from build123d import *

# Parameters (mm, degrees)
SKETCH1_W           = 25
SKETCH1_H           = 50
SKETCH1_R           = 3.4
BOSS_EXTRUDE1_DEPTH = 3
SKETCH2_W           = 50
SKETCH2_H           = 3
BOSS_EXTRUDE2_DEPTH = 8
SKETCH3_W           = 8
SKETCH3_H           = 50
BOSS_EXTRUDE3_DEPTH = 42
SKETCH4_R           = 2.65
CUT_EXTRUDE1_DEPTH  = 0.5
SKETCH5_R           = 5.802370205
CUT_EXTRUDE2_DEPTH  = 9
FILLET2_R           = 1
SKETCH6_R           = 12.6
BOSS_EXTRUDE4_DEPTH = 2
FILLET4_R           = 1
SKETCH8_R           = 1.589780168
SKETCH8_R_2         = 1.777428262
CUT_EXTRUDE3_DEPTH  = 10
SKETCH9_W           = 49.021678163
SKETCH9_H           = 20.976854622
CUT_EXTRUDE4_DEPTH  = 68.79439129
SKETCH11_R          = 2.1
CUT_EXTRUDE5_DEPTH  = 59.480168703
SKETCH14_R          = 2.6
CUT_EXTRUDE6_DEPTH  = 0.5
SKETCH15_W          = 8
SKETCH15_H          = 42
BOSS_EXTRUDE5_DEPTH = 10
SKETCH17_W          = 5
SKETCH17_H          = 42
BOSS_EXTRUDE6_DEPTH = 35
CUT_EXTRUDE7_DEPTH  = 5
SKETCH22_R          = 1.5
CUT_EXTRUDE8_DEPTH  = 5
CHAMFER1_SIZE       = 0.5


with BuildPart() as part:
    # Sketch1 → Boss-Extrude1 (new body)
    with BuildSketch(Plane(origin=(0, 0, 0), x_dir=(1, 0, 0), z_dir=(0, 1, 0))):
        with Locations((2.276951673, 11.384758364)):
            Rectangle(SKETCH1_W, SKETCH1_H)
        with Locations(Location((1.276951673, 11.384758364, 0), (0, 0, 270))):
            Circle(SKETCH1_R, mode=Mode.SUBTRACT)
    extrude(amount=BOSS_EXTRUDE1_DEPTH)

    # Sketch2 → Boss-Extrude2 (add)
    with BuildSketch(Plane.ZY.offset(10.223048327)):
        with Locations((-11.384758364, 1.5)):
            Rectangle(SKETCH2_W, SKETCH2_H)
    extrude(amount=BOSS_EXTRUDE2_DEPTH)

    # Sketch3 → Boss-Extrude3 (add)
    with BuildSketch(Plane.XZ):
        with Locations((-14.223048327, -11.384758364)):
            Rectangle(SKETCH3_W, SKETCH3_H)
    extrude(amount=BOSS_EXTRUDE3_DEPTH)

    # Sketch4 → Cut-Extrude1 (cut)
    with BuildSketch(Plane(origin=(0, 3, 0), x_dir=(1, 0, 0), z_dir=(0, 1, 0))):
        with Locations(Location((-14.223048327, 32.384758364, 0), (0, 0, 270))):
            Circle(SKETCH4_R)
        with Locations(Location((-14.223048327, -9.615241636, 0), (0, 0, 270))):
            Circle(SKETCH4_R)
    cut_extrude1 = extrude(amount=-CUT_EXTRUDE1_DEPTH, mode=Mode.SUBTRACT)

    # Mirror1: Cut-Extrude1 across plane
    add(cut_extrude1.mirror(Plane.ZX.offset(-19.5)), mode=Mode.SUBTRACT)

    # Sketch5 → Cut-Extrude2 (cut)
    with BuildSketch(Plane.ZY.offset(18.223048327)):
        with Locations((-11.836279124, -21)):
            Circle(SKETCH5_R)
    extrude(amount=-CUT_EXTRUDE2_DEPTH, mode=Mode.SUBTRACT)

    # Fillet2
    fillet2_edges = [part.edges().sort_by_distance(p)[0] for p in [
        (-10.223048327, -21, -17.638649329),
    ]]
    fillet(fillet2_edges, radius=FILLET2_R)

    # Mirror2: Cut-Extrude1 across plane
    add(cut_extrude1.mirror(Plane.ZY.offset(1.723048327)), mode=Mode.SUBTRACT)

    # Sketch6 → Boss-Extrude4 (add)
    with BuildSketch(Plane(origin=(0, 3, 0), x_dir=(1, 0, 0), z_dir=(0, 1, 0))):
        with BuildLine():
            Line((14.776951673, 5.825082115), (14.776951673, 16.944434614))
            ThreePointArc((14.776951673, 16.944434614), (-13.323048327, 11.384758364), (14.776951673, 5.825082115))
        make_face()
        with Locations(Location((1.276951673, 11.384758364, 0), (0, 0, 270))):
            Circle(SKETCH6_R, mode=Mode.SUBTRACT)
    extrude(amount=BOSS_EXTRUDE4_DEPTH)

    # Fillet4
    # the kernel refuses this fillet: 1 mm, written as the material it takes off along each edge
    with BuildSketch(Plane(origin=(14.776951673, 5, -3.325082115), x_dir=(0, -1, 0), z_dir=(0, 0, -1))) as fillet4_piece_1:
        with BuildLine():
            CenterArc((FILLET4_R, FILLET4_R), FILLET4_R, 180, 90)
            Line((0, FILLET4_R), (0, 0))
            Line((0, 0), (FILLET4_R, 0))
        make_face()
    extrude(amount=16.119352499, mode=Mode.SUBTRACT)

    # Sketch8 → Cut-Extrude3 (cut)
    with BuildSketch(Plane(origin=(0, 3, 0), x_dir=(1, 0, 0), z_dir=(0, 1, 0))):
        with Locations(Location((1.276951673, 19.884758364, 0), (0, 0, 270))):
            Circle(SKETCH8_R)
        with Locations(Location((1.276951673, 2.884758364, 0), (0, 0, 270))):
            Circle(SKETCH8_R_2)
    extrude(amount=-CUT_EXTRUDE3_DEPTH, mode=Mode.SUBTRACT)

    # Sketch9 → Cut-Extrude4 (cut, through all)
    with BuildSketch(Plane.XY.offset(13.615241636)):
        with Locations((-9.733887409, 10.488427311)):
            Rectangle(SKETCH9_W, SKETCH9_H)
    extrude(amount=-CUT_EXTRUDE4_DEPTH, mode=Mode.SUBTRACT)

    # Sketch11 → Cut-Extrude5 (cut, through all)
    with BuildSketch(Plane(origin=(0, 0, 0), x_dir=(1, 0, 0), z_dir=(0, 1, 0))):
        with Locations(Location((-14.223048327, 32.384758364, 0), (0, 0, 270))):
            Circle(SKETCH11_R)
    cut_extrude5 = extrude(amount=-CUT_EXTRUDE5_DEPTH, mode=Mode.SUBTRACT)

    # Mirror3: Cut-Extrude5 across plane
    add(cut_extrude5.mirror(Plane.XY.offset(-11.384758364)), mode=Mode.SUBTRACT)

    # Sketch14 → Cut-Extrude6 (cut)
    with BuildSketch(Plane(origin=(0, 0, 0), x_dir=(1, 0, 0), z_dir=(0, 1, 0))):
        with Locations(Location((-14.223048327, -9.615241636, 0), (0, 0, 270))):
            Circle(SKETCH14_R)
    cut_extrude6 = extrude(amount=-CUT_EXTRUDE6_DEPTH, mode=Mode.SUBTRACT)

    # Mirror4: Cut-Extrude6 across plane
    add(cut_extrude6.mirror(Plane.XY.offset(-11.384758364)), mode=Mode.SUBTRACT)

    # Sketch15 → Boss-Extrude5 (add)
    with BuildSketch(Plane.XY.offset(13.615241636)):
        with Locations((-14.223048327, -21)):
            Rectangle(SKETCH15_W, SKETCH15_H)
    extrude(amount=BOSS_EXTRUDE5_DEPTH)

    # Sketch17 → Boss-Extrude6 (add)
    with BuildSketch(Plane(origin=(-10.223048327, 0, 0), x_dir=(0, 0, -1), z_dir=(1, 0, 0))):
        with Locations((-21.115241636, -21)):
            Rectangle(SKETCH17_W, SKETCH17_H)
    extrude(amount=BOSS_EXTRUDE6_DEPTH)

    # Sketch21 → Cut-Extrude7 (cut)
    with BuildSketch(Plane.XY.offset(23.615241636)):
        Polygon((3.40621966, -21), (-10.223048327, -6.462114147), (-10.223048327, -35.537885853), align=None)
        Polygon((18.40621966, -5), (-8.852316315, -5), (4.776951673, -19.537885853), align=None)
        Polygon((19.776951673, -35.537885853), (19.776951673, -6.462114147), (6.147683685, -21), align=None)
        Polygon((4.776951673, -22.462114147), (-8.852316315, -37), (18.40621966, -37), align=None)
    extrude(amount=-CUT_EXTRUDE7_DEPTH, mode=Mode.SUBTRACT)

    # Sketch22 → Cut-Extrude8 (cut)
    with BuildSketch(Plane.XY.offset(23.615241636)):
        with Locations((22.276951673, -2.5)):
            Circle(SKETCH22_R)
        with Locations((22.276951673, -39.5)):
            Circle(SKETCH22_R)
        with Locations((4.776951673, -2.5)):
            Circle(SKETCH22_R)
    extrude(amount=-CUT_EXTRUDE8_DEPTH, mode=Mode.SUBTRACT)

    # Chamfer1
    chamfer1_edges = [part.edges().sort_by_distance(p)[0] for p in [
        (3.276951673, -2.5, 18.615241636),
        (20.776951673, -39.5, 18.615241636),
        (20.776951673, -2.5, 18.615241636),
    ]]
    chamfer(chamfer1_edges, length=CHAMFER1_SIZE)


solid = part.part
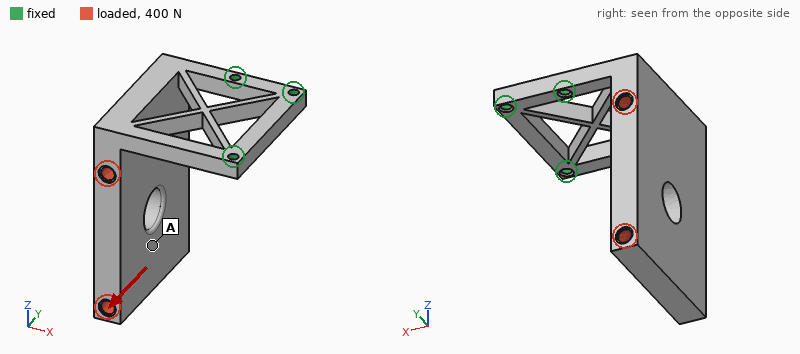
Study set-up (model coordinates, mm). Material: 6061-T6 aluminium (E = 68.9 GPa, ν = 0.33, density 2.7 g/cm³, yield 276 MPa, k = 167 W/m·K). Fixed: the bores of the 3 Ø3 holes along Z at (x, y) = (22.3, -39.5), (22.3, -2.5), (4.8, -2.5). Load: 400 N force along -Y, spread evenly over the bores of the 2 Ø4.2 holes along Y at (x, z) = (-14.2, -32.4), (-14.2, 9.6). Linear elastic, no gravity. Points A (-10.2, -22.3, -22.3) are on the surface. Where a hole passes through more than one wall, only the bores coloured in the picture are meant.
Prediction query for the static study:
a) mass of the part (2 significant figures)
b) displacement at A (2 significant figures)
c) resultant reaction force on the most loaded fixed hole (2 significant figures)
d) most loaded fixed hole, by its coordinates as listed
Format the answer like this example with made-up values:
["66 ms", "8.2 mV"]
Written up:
["58 g", "0.55 mm", "450 N", "(22.3, -39.5)"]
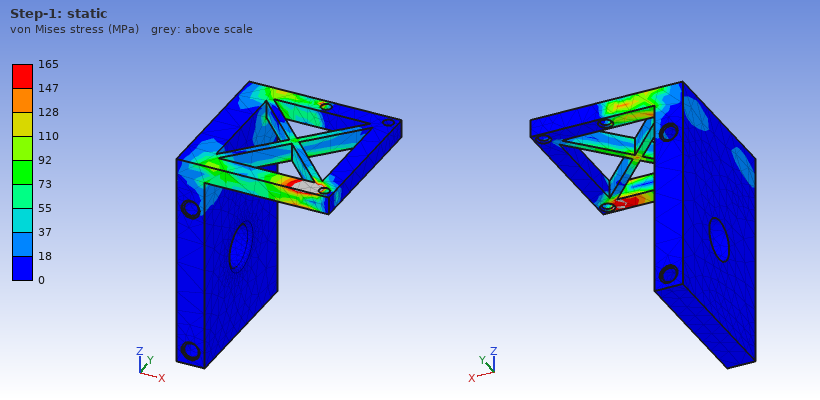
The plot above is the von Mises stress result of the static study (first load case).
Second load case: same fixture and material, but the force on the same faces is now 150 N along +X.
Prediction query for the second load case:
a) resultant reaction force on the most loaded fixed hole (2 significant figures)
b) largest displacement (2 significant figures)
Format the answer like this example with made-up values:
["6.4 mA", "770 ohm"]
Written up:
["80 N", "0.82 mm"]
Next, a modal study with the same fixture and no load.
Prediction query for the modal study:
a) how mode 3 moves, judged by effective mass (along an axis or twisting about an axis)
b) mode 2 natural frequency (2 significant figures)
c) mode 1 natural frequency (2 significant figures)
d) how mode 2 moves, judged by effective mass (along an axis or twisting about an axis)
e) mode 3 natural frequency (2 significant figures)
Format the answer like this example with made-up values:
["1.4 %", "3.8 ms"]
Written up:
["along Z", "810 Hz", "390 Hz", "along Y", "2200 Hz"]
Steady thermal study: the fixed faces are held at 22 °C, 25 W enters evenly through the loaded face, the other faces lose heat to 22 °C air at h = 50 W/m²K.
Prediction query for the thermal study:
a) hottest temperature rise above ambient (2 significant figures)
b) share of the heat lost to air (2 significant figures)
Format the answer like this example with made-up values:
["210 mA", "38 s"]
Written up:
["40 K", "51 %"]
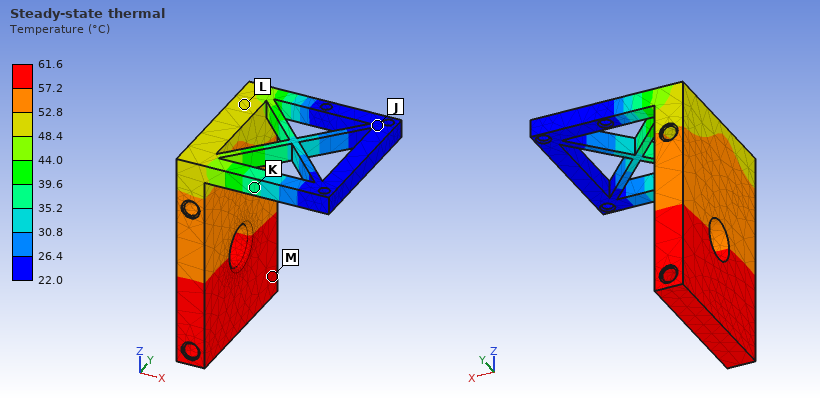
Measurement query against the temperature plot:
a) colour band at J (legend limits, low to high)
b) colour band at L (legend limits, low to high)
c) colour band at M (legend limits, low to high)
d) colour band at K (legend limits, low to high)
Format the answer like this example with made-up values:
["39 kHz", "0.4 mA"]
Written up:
["22.0 to 26.4 °C", "48.4 to 52.8 °C", "57.2 to 61.6 °C", "35.2 to 39.6 °C"]
